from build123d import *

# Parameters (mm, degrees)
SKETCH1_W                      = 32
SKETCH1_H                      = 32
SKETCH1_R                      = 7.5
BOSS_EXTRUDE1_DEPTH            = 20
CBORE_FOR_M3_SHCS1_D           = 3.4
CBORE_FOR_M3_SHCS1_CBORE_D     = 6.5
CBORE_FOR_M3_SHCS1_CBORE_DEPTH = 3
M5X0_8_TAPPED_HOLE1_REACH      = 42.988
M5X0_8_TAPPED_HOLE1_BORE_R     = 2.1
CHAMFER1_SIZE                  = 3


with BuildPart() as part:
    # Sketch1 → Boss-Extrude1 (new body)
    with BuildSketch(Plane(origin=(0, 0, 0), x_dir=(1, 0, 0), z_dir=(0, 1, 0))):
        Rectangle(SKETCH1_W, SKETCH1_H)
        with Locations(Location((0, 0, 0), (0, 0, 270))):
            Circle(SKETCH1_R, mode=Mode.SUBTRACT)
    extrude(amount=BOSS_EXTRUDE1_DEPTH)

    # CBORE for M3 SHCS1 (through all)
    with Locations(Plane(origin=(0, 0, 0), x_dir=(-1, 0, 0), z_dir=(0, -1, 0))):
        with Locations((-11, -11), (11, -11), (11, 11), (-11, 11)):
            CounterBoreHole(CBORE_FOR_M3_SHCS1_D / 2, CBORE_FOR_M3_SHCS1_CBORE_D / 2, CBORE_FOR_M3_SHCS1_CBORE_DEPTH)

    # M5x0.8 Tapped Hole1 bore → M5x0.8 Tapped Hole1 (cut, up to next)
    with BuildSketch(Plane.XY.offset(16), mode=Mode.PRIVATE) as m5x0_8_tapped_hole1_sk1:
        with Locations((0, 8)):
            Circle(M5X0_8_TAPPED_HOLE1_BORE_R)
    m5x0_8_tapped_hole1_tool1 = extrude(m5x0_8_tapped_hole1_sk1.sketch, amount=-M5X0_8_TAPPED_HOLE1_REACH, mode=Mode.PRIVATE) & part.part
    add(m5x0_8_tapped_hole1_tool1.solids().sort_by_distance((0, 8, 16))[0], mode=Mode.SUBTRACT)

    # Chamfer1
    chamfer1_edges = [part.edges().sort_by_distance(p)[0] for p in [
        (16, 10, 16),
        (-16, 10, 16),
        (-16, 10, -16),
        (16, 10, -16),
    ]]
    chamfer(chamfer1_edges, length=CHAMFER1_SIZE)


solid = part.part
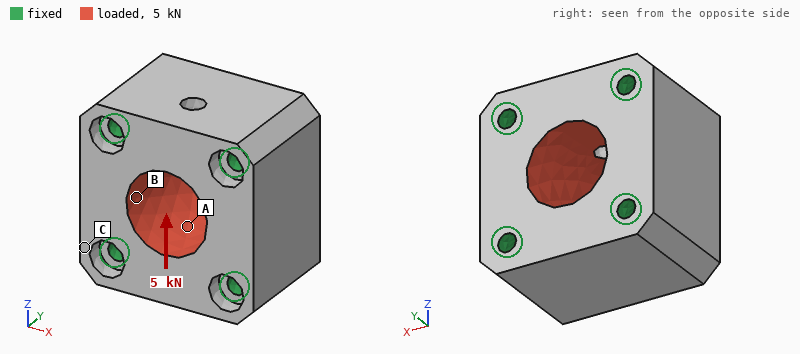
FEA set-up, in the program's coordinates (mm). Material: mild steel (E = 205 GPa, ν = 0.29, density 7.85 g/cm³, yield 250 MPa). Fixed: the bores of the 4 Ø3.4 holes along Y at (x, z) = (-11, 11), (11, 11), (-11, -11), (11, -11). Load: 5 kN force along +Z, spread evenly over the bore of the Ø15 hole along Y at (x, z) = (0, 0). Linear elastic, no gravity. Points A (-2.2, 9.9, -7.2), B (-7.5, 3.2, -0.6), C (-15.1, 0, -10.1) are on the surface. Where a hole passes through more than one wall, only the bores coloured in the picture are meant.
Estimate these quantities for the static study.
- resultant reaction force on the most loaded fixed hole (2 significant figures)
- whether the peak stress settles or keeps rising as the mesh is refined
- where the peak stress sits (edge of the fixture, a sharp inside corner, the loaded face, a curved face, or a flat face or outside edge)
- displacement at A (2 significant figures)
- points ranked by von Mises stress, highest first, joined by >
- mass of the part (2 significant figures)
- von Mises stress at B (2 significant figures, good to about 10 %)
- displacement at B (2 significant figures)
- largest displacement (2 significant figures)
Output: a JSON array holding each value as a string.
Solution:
["1.3 kN", "keeps rising", "edge of the fixture", "0.57 µm", "B > A > C", "120 g", "10 MPa", "0.39 µm", "0.77 µm"]
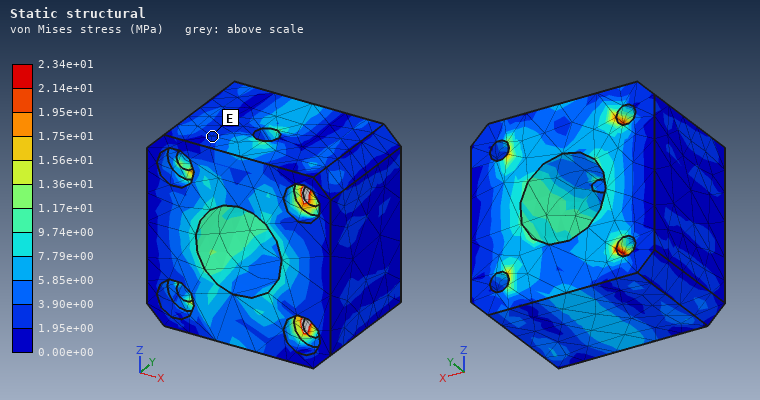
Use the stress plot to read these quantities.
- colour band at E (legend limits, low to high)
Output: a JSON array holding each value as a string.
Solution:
["1.95e+00 to 3.90e+00 MPa"]
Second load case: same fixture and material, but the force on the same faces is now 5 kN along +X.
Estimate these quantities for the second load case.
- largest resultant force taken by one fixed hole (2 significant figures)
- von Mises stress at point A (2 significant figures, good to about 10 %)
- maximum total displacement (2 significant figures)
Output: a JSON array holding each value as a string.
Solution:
["1.3 kN", "10 MPa", "0.78 µm"]
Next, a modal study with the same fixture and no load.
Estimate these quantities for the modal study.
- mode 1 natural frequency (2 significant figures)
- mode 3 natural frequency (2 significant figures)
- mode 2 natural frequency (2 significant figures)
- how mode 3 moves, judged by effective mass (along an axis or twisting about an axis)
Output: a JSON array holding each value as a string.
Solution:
["46 kHz", "61 kHz", "58 kHz", "along X"]
